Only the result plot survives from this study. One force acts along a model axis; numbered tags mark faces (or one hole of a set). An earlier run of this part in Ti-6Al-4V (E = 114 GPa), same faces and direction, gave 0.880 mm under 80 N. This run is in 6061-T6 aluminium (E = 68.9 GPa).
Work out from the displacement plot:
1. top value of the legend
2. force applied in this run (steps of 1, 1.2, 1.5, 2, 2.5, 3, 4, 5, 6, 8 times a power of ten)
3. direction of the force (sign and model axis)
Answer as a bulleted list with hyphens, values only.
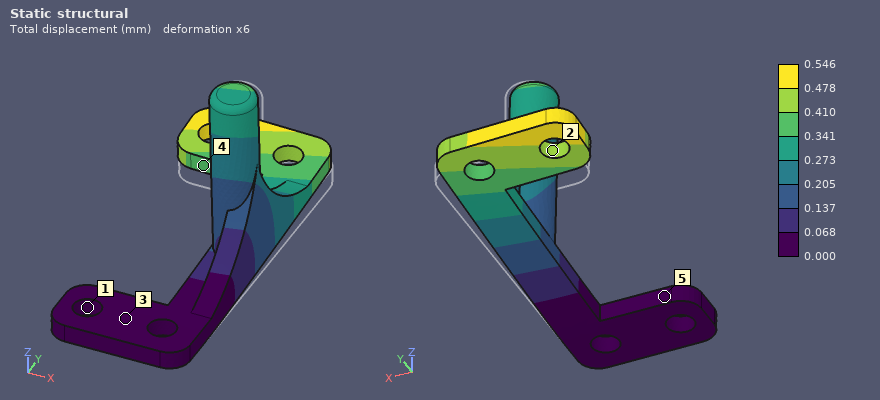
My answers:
- 0.546 mm
- 30 N
- +Z
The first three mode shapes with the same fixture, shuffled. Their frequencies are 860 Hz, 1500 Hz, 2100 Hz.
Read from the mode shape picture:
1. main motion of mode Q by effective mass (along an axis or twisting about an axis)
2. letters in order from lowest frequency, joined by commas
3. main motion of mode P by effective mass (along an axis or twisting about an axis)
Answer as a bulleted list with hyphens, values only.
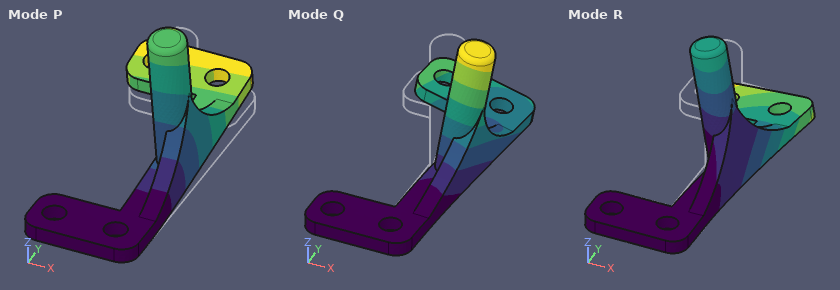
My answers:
- along X
- P, Q, R
- along Z
